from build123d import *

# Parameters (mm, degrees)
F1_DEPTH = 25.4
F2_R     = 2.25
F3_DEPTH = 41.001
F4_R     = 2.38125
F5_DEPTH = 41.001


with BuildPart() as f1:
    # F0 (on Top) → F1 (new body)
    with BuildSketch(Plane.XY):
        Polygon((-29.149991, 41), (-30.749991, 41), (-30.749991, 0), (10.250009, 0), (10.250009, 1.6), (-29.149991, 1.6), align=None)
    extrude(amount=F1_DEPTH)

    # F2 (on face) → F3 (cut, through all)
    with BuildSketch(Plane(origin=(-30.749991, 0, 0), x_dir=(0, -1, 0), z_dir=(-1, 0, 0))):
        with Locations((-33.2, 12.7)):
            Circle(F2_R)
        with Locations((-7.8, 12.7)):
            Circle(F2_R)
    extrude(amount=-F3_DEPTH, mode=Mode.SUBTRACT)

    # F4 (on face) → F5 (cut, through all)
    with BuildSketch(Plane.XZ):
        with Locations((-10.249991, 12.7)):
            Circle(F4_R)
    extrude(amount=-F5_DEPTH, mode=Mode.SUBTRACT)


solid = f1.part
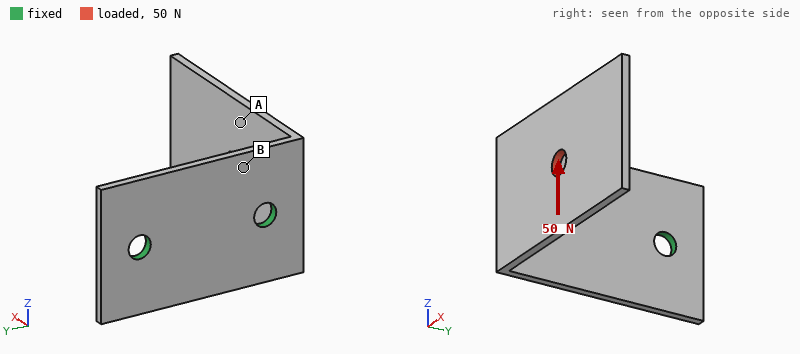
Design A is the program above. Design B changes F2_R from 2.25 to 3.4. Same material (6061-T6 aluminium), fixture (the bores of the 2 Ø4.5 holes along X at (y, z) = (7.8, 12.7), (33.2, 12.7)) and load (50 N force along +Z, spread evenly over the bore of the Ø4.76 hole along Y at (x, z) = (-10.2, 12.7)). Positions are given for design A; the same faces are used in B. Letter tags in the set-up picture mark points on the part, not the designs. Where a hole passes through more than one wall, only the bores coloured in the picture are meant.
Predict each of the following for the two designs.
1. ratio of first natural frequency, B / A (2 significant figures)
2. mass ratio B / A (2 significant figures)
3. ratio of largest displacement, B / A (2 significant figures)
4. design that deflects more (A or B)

1.1
0.98
0.64
A
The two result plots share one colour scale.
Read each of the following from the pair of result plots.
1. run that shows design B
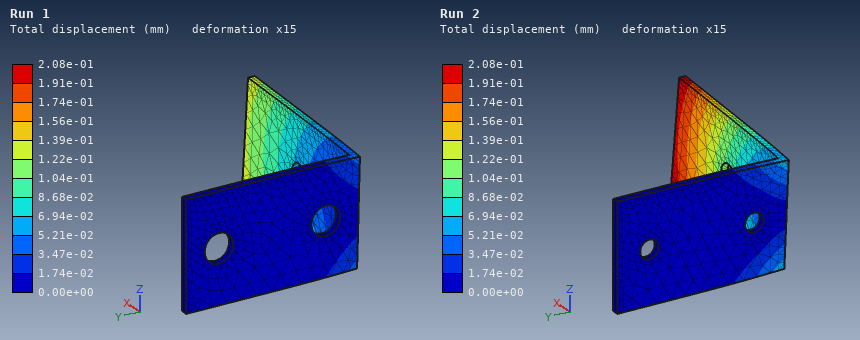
Run 1
